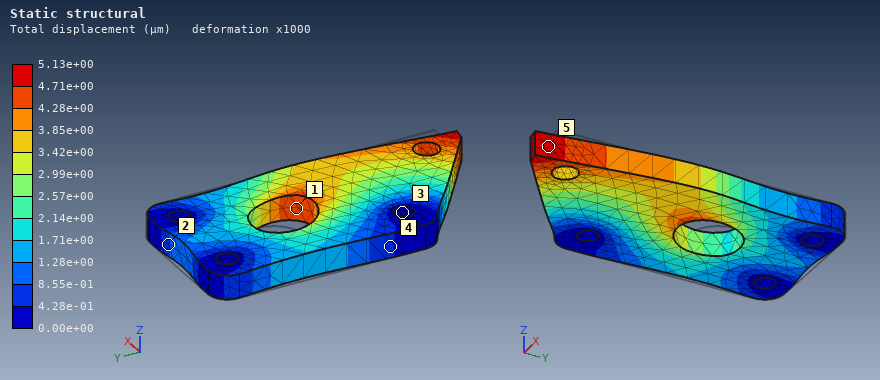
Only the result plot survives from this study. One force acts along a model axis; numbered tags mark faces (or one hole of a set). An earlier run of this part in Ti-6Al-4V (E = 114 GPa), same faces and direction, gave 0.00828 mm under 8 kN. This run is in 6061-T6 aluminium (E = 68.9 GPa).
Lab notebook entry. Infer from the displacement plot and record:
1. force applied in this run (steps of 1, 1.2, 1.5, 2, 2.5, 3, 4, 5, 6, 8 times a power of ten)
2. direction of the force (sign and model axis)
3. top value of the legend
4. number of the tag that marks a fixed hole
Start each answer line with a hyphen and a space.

- 3 kN
- -Y
- 5.13e+00 µm
- 3
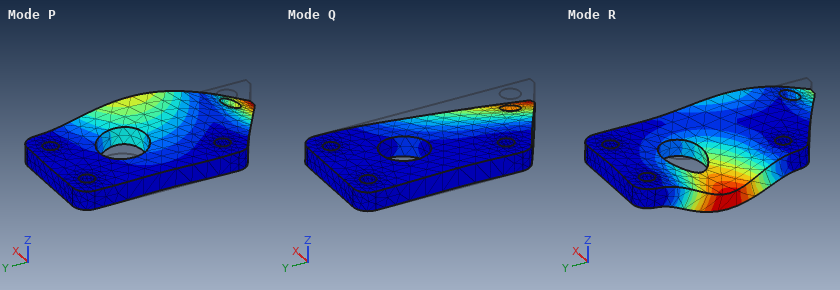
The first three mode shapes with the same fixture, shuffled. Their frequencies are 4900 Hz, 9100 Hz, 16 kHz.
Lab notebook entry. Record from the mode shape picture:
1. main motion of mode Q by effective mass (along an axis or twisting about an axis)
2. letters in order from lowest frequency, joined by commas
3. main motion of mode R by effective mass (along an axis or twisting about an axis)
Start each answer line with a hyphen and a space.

- along Z
- Q, P, R
- along Z
